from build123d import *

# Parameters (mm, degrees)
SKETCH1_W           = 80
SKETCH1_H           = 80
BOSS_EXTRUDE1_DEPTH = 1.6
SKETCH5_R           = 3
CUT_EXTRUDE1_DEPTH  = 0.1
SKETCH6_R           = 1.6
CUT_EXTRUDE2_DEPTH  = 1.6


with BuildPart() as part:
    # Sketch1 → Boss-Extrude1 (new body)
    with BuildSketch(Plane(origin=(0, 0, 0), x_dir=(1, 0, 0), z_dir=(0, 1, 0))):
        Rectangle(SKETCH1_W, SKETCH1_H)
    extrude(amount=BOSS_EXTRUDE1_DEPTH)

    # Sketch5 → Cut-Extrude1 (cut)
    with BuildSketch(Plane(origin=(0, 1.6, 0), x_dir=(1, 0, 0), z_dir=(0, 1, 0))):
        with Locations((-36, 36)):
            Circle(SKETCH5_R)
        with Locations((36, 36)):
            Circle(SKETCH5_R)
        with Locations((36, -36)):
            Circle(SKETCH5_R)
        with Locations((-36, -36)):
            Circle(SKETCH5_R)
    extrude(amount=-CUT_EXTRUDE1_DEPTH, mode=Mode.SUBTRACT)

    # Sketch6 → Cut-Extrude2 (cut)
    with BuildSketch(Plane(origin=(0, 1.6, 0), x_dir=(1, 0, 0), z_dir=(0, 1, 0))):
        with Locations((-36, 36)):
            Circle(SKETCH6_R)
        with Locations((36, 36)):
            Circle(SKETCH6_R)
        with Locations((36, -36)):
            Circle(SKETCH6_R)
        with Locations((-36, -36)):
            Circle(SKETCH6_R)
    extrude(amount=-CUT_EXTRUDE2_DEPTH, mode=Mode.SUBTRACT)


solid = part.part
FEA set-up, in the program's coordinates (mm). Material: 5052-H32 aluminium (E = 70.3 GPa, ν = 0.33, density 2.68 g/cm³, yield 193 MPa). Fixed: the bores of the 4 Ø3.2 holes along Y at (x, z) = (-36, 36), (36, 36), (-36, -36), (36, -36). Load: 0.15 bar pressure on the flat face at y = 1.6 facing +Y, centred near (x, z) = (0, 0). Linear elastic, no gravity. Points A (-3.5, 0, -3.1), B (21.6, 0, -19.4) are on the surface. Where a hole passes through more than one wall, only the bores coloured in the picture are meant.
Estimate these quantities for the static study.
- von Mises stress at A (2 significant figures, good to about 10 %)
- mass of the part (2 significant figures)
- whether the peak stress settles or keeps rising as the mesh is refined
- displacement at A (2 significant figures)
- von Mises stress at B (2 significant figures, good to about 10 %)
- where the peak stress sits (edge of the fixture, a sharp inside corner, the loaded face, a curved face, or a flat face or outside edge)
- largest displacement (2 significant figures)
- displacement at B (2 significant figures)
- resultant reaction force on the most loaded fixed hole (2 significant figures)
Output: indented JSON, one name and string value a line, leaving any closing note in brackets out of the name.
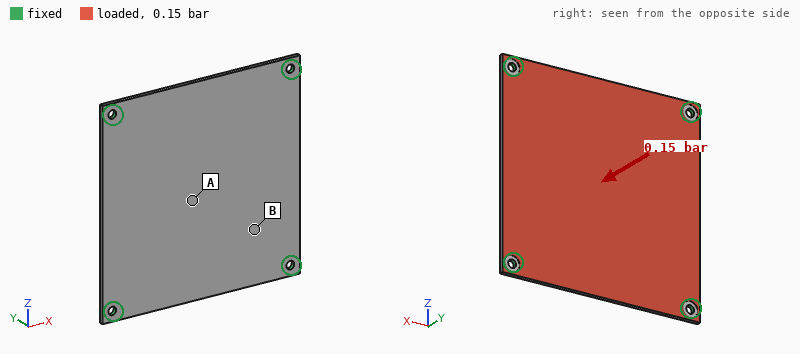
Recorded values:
{
  "von Mises stress at A": "11 MPa",
  "mass of the part": "27 g",
  "whether the peak stress settles or keeps rising as the mesh is refined": "keeps rising",
  "displacement at A": "0.12 mm",
  "von Mises stress at B": "5.3 MPa",
  "where the peak stress sits": "edge of the fixture",
  "largest displacement": "0.13 mm",
  "displacement at B": "0.072 mm",
  "resultant reaction force on the most loaded fixed hole": "24 N"
}
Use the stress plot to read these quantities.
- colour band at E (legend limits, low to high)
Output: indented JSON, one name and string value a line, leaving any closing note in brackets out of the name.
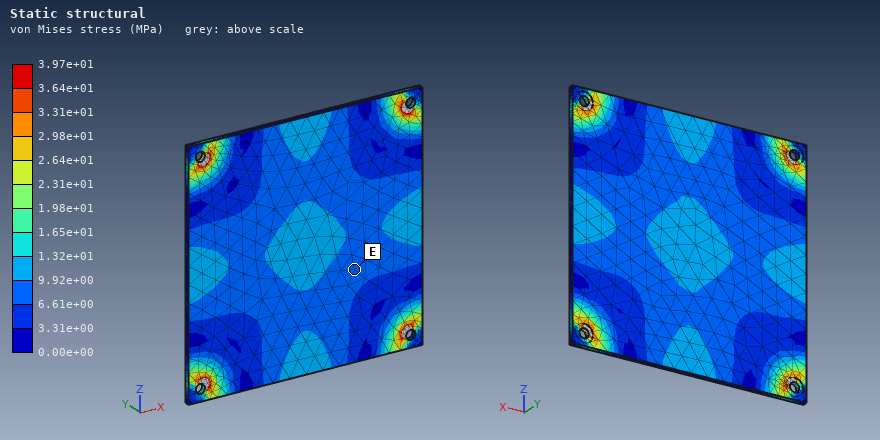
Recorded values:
{
  "colour band at E": "6.61e+00 to 9.92e+00 MPa"
}
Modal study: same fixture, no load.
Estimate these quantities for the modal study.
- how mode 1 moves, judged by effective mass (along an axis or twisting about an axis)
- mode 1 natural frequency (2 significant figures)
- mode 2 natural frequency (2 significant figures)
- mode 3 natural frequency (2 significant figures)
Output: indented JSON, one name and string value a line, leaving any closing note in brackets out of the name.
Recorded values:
{
  "how mode 1 moves, judged by effective mass": "along Y",
  "mode 1 natural frequency": "1000 Hz",
  "mode 2 natural frequency": "1800 Hz",
  "mode 3 natural frequency": "1800 Hz"
}
